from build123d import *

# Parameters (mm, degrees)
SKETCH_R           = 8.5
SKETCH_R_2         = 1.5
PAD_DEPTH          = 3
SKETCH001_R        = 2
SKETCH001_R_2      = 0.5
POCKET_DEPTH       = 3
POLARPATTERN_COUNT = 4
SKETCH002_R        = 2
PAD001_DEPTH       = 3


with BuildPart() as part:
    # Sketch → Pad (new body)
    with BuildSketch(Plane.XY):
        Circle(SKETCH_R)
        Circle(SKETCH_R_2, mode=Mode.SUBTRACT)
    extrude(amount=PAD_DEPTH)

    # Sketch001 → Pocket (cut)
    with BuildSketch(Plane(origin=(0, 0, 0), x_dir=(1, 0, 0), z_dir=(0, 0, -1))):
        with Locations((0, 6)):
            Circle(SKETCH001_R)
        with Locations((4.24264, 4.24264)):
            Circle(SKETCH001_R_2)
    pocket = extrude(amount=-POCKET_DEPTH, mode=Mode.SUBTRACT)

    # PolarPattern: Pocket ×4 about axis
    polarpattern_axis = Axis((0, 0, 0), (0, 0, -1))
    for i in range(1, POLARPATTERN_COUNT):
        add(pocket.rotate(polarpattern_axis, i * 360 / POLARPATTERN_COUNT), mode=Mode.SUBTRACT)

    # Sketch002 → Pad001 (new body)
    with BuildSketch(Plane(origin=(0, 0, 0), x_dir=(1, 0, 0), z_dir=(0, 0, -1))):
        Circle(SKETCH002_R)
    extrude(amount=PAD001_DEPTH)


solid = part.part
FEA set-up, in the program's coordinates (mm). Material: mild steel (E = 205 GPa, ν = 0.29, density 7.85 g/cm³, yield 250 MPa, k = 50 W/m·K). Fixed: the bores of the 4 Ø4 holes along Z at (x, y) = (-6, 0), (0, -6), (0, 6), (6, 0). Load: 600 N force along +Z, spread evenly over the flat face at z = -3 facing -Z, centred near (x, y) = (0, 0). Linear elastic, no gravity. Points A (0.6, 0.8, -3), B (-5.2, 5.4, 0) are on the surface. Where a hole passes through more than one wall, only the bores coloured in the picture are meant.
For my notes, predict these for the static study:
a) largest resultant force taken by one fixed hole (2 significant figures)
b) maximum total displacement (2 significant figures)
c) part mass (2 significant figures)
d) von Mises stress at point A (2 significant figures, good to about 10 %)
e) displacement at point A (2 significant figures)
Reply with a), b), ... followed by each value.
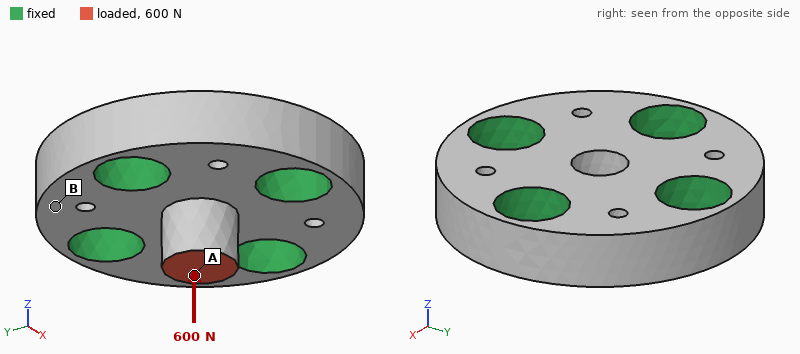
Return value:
a) 170 N
b) 1.7 µm
c) 4.2 g
d) 49 MPa
e) 1.7 µm
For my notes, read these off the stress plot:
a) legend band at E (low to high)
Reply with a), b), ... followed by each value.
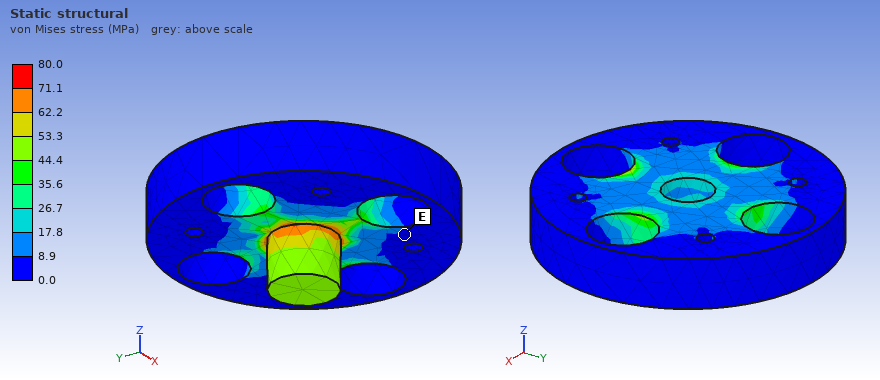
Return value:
a) 0.0 to 8.9 MPa
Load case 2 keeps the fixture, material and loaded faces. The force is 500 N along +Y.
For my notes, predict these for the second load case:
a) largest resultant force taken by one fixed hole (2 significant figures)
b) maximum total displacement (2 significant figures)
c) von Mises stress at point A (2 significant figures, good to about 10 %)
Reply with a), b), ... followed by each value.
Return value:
a) 340 N
b) 7.6 µm
c) 87 MPa
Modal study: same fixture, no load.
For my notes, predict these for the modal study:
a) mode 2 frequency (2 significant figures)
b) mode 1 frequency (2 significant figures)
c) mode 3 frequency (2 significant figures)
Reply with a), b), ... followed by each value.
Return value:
a) 120 kHz
b) 120 kHz
c) 170 kHz
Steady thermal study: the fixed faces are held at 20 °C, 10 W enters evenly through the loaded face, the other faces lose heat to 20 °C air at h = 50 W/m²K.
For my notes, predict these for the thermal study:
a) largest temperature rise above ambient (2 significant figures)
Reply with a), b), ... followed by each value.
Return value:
a) 80 K
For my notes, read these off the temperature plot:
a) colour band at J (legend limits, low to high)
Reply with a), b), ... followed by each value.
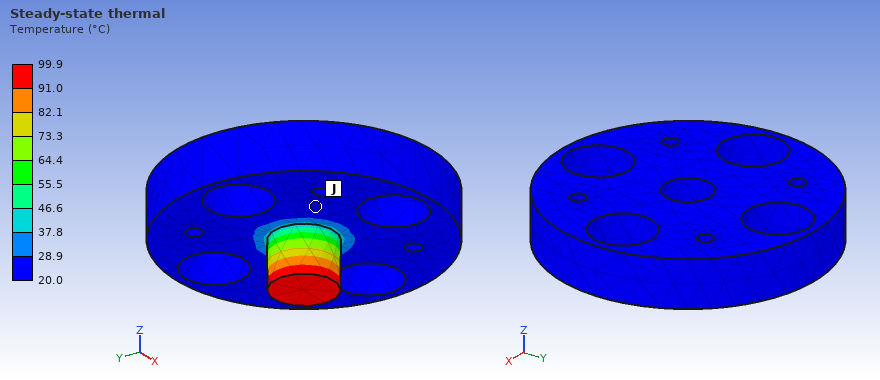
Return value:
a) 20.0 to 28.9 °C
